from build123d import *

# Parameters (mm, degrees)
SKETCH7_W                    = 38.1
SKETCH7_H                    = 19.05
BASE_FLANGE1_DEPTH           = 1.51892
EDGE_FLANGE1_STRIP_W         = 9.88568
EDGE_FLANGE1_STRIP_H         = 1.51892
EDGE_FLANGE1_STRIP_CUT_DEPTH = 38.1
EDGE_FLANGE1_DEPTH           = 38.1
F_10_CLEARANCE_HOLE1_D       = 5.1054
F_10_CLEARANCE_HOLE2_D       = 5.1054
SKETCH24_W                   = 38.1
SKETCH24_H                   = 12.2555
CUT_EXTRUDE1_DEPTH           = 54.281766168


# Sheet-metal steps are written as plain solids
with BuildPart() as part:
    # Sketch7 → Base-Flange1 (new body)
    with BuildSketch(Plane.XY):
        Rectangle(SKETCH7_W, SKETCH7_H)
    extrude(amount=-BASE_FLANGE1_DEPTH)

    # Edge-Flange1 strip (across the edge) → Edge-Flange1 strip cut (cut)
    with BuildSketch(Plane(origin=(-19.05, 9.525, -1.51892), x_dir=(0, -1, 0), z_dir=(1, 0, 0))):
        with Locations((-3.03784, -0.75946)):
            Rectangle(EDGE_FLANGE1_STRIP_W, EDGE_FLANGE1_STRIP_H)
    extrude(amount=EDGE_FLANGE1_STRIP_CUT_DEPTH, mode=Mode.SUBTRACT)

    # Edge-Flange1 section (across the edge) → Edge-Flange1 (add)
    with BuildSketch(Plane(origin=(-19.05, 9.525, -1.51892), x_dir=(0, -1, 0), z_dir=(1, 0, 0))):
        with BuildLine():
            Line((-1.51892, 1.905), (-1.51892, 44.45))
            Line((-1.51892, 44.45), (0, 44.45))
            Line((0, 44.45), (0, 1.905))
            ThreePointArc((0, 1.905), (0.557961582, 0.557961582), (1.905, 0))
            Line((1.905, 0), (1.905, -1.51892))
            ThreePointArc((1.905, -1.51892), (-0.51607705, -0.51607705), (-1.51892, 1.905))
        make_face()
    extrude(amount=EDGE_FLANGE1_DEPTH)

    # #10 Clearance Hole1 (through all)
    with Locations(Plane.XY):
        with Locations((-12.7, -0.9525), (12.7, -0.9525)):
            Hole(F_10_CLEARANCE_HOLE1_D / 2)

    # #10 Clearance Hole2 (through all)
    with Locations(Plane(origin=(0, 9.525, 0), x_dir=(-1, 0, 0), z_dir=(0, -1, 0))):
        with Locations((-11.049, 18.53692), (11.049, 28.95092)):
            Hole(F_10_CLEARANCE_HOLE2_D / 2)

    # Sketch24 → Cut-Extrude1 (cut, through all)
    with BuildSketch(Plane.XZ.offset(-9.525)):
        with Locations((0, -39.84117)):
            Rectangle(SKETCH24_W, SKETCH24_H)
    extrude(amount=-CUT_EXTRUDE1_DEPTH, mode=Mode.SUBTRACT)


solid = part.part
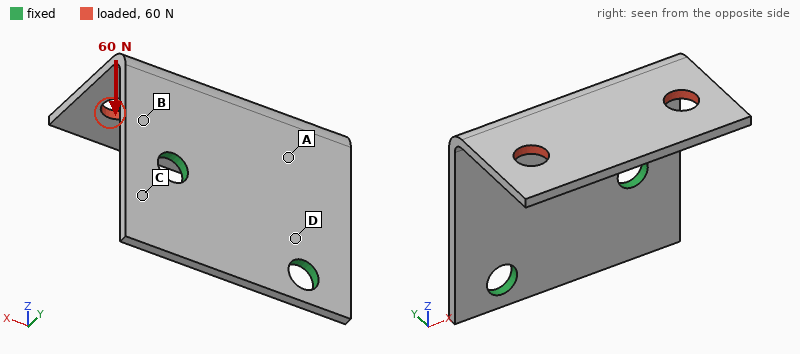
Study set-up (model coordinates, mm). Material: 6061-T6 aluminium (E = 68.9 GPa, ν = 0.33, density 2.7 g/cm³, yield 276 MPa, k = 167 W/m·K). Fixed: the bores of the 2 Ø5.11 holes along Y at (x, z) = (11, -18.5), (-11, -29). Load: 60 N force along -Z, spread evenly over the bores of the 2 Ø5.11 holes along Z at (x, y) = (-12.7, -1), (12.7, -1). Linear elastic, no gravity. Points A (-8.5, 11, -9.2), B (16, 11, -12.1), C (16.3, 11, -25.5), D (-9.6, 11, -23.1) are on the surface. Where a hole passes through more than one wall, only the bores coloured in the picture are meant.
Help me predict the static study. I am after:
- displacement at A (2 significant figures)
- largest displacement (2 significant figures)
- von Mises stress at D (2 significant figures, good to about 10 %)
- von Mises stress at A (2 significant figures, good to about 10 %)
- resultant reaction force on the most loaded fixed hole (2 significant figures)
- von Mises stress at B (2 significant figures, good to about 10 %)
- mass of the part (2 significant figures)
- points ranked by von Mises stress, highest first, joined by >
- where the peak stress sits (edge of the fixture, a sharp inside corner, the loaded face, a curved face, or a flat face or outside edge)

0.071 mm
0.43 mm
20 MPa
35 MPa
32 N
52 MPa
7.7 g
B > A > D > C
a flat face or outside edge
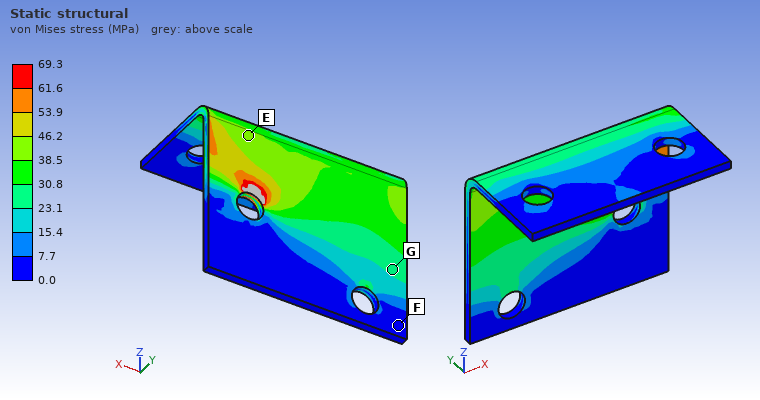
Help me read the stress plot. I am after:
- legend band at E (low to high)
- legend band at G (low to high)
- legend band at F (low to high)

38.5 to 46.2 MPa
23.1 to 30.8 MPa
0.0 to 7.7 MPa
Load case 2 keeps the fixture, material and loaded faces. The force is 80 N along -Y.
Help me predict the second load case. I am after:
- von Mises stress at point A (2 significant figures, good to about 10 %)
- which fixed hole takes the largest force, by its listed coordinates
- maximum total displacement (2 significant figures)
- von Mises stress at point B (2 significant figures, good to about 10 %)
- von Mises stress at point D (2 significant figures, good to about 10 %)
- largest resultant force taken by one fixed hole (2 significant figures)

33 MPa
(11, -18.5)
0.57 mm
83 MPa
61 MPa
67 N
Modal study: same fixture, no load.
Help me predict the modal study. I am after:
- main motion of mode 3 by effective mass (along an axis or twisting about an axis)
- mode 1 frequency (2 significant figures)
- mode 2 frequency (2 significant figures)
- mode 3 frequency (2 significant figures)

along Y
1100 Hz
1900 Hz
3200 Hz
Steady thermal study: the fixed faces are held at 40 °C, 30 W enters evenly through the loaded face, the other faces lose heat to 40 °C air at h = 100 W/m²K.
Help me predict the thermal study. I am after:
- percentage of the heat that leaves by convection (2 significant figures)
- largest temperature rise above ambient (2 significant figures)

42 %
79 K
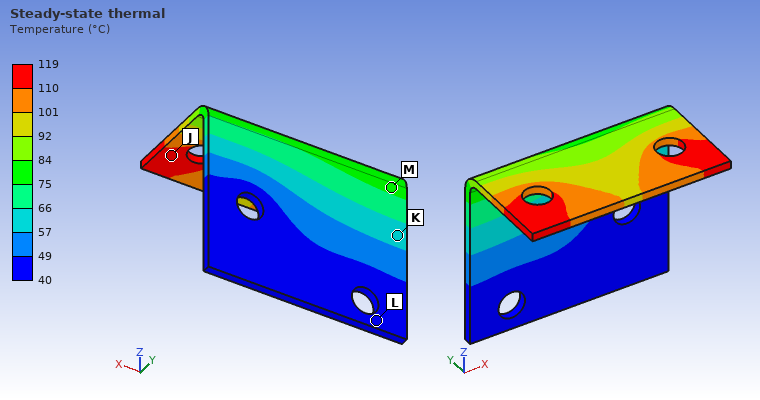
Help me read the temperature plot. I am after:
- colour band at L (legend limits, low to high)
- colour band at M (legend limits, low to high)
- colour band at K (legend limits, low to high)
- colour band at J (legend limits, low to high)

40 to 49 °C
75 to 84 °C
57 to 66 °C
110 to 119 °C
